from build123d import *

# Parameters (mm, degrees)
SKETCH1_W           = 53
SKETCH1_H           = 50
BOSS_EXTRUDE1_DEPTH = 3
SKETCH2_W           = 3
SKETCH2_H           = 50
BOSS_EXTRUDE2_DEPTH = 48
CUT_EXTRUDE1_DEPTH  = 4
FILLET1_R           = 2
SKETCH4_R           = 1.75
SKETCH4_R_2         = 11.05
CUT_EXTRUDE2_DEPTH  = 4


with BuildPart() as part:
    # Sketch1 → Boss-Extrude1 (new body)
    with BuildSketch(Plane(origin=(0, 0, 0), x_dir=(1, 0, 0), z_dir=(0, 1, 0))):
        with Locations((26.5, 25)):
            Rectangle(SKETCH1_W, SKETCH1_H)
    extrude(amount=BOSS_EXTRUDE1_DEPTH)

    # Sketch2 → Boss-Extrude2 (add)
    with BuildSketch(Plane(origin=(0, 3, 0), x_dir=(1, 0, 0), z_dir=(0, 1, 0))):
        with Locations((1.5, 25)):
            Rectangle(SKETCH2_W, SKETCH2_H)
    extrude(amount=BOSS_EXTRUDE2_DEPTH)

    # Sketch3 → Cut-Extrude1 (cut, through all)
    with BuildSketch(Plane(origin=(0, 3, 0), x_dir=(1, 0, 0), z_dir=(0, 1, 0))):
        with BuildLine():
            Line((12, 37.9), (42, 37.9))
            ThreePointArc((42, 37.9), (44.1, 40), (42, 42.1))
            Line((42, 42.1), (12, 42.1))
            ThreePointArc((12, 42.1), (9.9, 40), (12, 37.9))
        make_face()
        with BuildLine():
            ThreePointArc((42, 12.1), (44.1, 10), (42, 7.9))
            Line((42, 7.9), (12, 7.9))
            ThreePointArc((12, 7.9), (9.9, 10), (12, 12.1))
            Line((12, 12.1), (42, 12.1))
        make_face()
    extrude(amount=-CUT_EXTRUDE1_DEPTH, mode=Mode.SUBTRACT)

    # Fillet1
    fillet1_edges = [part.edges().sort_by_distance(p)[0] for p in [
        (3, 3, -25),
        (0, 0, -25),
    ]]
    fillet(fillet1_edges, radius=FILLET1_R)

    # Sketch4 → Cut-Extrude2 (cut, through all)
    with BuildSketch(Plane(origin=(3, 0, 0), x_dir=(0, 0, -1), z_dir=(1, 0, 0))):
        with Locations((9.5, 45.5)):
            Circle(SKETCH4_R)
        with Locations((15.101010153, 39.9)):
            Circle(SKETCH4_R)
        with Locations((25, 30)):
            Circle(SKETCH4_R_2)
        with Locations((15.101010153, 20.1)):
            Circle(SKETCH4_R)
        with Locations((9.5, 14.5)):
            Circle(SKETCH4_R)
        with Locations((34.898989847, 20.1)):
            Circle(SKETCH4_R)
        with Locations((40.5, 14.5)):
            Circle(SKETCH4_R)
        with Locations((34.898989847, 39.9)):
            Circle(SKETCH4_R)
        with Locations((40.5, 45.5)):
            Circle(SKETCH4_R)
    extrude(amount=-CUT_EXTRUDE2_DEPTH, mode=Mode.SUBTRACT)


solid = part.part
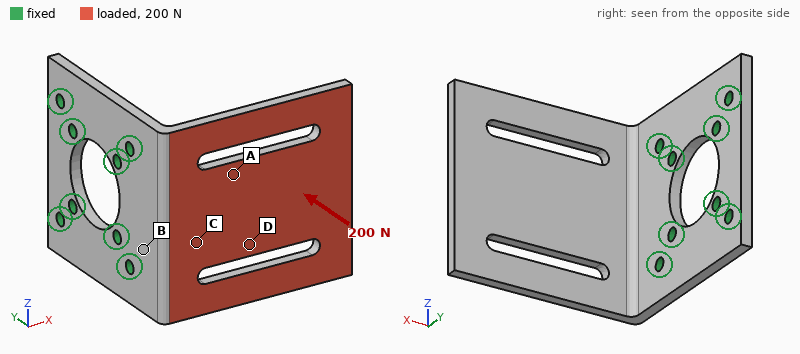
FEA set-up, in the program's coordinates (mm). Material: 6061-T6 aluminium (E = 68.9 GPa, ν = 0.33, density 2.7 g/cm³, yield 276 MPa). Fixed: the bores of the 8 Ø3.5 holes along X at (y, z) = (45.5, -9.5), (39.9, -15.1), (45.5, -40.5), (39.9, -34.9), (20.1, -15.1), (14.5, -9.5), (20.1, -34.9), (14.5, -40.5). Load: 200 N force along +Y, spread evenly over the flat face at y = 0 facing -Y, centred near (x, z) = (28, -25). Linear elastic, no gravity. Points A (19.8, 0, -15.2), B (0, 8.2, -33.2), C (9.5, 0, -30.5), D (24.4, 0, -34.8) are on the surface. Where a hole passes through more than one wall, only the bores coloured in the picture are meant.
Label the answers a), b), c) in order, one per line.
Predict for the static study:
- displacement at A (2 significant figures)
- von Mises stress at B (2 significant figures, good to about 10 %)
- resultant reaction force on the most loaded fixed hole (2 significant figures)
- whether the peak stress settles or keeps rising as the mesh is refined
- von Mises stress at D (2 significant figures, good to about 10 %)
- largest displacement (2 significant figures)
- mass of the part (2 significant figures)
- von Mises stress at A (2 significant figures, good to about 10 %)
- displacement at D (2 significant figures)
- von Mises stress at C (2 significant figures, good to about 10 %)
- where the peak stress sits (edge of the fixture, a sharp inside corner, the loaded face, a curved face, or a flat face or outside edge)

a) 0.23 mm
b) 60 MPa
c) 140 N
d) keeps rising
e) 26 MPa
f) 0.83 mm
g) 35 g
h) 35 MPa
i) 0.30 mm
j) 50 MPa
k) edge of the fixture
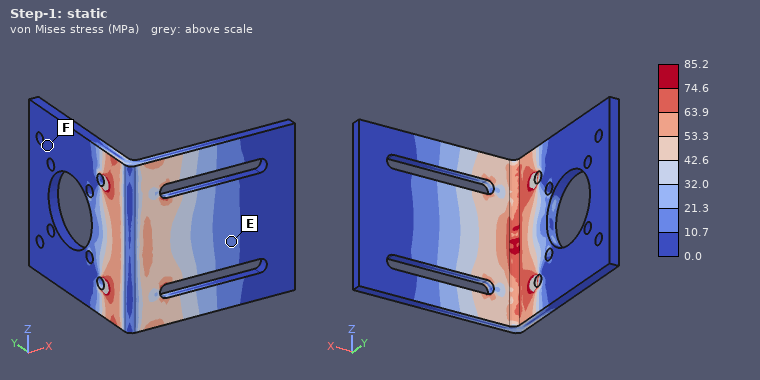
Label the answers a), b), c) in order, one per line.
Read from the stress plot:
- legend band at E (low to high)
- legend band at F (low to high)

a) 10.7 to 21.3 MPa
b) 0.0 to 10.7 MPa
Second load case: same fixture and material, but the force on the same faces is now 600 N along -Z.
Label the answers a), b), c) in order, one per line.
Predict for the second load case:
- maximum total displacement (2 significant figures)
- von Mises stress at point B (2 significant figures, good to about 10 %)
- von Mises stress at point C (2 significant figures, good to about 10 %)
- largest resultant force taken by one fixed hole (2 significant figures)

a) 0.22 mm
b) 38 MPa
c) 16 MPa
d) 620 N
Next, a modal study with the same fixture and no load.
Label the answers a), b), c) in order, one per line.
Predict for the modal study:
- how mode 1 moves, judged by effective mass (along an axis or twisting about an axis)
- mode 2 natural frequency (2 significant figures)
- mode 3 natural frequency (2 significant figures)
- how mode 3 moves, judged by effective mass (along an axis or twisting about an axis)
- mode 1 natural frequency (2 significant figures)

a) along Y
b) 1800 Hz
c) 2600 Hz
d) along Z
e) 700 Hz
